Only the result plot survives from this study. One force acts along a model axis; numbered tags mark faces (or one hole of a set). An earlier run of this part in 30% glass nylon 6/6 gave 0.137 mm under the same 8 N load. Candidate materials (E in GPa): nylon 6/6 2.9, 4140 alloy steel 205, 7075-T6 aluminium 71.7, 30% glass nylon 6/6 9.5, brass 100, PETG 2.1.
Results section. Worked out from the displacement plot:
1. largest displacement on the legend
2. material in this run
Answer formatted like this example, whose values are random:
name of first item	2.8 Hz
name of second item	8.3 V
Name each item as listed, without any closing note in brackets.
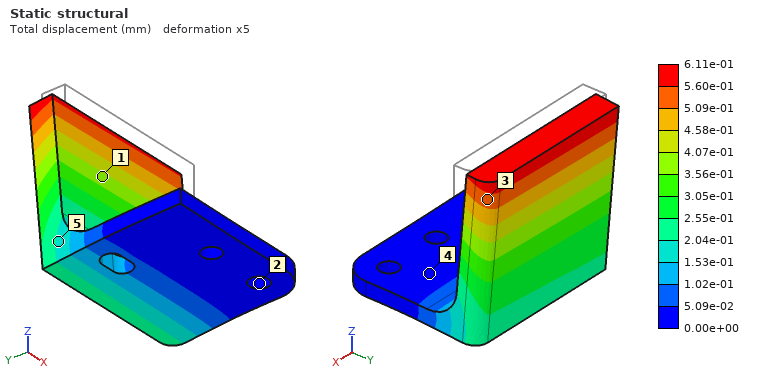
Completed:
largest displacement on the legend	6.11e-01 mm
material in this run	PETG
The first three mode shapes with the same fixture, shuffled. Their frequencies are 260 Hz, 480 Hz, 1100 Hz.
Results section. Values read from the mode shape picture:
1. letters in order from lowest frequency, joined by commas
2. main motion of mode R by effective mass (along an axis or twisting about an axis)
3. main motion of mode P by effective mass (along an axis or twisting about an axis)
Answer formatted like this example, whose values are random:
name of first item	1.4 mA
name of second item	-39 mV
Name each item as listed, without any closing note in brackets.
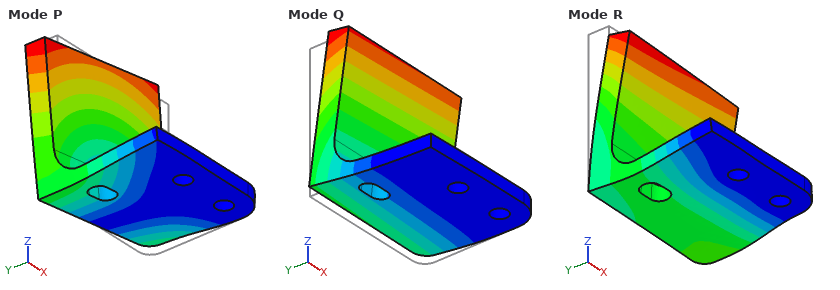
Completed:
letters in order from lowest frequency, joined by commas	Q, P, R
main motion of mode R by effective mass	along Z
main motion of mode P by effective mass	along X
